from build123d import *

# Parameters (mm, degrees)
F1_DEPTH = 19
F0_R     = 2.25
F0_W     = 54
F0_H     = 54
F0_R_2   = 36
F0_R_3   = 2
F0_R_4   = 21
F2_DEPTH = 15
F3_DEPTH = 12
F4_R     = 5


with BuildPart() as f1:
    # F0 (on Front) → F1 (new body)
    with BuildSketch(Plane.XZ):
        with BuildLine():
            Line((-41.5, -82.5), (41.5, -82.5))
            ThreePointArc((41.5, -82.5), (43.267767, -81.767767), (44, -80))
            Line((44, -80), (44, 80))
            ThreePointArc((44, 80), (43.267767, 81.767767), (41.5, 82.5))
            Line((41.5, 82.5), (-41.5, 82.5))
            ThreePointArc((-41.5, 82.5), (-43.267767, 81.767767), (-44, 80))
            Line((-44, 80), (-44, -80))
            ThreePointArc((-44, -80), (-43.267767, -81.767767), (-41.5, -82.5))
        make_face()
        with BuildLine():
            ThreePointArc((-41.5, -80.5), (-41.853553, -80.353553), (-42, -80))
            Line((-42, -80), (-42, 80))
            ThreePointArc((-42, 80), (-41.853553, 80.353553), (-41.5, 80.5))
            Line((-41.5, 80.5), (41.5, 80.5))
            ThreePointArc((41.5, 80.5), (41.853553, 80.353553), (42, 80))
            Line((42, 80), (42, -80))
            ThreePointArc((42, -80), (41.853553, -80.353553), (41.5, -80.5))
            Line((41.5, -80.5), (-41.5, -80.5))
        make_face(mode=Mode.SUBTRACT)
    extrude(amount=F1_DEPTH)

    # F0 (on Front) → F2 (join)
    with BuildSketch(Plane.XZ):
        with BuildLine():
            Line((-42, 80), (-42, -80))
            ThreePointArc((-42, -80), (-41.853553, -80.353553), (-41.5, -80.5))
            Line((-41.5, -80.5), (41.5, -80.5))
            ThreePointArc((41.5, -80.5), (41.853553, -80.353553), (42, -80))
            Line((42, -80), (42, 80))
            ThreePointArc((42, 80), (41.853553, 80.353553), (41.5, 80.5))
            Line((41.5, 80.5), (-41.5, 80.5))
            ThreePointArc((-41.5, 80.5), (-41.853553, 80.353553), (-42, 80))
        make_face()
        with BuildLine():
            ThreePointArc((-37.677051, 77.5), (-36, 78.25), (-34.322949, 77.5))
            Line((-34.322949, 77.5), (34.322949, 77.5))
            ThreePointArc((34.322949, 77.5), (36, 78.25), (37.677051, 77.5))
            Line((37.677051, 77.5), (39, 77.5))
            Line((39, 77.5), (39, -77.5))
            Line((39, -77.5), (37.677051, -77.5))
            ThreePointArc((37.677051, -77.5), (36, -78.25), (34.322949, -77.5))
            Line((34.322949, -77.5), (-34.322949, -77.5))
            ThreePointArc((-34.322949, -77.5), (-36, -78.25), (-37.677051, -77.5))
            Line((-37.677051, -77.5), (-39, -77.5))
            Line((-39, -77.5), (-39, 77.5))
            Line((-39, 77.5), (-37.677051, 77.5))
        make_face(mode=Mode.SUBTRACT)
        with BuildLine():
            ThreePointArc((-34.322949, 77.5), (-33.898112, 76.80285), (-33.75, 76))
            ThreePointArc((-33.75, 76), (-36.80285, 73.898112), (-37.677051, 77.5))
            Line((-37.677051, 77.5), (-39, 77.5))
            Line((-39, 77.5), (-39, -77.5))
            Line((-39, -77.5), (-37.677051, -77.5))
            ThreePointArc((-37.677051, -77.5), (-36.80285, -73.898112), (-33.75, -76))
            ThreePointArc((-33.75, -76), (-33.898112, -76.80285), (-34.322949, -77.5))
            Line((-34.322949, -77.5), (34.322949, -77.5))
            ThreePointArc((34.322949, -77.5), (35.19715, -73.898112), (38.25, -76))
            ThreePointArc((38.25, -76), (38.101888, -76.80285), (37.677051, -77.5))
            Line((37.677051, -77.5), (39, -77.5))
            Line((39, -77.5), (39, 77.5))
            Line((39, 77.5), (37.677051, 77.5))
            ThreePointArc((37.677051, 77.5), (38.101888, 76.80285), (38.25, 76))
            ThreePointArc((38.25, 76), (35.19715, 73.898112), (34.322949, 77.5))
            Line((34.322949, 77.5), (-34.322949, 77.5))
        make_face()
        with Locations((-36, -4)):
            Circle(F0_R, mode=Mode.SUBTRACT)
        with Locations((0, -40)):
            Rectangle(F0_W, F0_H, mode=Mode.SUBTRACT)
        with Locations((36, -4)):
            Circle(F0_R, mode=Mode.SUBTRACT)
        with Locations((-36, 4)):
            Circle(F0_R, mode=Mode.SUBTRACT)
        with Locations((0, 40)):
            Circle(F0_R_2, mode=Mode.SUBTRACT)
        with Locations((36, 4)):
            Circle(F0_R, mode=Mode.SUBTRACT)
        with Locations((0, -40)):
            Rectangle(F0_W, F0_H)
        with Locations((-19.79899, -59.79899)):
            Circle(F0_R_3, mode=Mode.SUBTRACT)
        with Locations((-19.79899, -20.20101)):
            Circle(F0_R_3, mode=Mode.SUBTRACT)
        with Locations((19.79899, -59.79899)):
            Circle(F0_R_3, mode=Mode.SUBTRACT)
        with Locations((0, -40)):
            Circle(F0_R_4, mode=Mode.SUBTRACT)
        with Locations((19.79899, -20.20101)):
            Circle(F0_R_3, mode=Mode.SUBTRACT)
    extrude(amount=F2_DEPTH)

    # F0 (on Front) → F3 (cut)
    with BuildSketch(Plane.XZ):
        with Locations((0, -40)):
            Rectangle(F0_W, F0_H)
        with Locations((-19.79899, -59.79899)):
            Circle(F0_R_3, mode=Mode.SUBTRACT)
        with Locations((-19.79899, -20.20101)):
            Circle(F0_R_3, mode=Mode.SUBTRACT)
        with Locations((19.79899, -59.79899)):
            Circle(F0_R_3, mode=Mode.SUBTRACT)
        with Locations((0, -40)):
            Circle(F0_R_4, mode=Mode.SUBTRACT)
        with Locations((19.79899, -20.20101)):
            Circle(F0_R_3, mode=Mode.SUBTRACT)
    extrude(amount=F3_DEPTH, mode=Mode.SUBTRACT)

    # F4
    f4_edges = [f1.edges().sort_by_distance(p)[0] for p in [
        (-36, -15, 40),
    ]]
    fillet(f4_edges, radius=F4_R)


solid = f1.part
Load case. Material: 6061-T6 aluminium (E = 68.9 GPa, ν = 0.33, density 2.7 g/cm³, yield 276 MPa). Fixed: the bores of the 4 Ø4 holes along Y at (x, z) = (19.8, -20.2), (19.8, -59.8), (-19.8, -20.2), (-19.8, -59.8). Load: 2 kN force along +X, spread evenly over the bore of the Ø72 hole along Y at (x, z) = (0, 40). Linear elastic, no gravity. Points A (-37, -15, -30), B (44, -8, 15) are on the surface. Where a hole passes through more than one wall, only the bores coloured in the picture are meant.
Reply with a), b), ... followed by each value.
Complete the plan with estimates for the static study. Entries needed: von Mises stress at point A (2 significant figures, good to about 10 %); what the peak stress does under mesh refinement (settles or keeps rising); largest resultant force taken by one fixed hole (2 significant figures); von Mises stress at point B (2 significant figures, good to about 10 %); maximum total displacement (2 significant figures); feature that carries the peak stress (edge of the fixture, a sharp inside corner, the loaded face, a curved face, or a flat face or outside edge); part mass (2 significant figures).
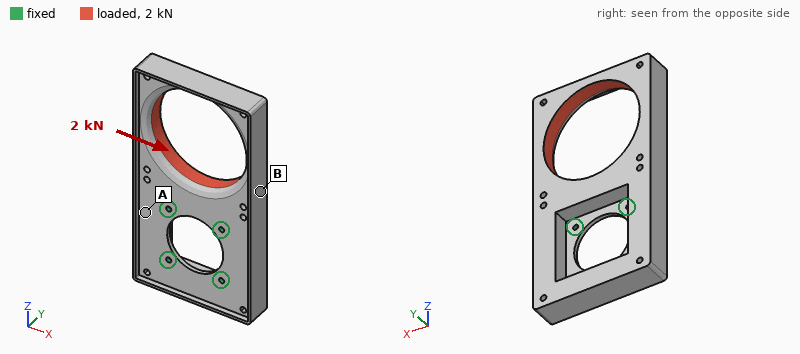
a) 9.0 MPa
b) keeps rising
c) 1.9 kN
d) 25 MPa
e) 0.13 mm
f) edge of the fixture
g) 320 g
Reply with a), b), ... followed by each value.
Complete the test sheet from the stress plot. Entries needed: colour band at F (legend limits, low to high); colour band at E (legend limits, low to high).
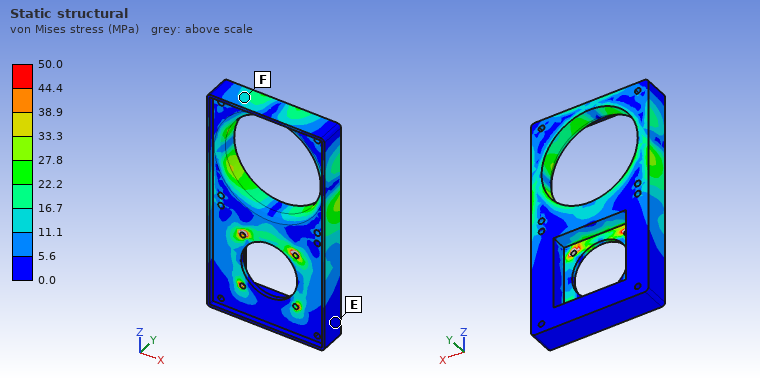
a) 11.1 to 16.7 MPa
b) 0.0 to 5.6 MPa
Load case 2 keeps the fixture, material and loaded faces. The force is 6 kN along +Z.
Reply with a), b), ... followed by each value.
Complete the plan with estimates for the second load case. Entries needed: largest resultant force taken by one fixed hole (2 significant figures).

a) 1.7 kN
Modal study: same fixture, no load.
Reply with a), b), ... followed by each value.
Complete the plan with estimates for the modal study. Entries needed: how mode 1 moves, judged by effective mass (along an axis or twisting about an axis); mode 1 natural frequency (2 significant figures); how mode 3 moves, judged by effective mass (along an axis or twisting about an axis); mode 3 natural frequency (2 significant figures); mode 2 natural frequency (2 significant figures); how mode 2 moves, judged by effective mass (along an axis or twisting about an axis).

a) along Y
b) 760 Hz
c) along X
d) 1800 Hz
e) 1400 Hz
f) twisting about Z
